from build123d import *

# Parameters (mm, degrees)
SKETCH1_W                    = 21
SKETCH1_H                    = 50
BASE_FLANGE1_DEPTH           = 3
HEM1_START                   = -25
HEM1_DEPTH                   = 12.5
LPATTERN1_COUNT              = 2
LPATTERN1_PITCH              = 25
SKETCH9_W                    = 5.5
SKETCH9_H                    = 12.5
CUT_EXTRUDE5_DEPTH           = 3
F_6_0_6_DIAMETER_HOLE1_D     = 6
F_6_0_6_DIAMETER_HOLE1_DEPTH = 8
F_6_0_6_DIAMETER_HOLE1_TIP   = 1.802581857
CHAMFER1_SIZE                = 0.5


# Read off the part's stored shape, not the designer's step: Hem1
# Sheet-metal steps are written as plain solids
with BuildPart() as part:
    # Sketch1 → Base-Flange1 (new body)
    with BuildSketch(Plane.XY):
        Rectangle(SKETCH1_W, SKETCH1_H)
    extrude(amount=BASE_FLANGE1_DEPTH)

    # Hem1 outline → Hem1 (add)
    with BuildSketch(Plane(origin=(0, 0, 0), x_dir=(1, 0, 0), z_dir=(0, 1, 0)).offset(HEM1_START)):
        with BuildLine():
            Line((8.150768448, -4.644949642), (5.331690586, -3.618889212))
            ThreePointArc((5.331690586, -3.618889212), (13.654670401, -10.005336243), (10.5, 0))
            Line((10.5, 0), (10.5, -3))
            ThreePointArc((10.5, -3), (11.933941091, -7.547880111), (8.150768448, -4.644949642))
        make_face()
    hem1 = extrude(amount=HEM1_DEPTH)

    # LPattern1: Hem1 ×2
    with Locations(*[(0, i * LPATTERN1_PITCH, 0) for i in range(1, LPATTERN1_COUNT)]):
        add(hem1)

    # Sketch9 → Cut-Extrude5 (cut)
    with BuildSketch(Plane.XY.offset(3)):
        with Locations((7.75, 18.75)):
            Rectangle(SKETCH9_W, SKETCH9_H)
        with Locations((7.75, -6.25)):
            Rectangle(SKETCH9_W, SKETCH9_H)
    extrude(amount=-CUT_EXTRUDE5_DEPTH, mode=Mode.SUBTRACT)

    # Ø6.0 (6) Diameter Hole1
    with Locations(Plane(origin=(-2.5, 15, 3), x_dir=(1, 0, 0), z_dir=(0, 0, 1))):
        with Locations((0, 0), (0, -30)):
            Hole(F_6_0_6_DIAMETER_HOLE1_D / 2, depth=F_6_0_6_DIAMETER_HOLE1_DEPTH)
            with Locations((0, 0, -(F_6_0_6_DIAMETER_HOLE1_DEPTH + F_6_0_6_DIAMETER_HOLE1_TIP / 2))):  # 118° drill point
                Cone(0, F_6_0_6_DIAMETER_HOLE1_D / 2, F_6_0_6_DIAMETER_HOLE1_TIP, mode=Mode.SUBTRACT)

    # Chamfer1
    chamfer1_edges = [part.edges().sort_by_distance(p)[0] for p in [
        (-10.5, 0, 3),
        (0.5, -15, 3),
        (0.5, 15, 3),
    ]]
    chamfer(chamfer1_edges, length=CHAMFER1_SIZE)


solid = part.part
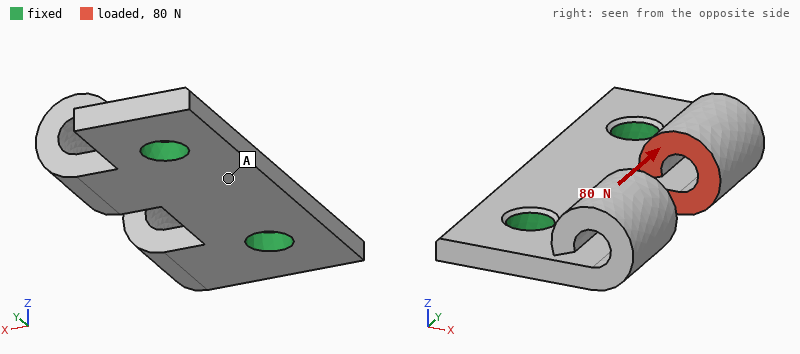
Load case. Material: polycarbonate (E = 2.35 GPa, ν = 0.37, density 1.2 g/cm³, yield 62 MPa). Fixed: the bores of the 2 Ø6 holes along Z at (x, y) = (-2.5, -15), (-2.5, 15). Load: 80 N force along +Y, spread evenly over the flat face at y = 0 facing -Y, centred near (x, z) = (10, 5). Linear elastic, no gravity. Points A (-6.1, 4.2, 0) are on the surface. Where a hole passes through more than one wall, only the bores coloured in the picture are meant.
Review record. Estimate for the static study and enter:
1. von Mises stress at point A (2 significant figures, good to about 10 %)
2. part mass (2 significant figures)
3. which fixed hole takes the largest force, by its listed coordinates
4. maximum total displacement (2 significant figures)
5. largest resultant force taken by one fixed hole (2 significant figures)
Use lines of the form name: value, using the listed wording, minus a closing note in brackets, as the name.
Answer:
von Mises stress at point A: 2.7 MPa
part mass: 4.9 g
which fixed hole takes the largest force, by its listed coordinates: (-2.5, 15)
maximum total displacement: 0.56 mm
largest resultant force taken by one fixed hole: 63 N
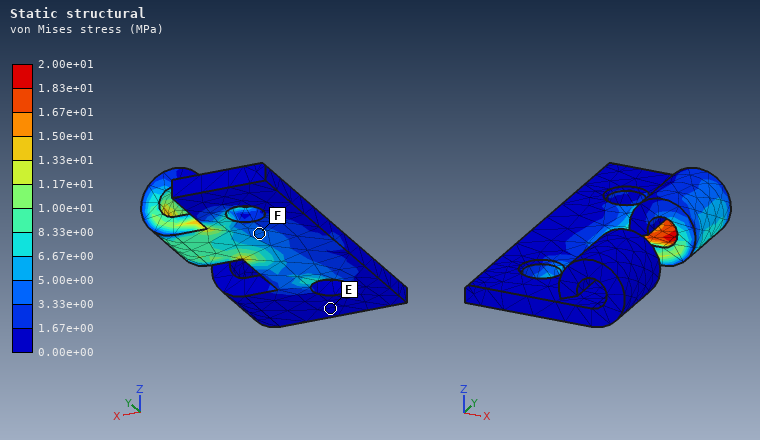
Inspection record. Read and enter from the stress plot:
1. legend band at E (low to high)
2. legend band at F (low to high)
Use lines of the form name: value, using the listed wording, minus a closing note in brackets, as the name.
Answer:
legend band at E: 0.00e+00 to 1.67e+00 MPa
legend band at F: 3.33e+00 to 5.00e+00 MPa
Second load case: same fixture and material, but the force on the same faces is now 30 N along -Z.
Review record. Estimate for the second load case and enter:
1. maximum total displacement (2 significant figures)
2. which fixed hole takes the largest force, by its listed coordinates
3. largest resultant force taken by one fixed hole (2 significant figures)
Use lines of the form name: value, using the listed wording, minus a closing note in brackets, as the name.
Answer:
maximum total displacement: 0.64 mm
which fixed hole takes the largest force, by its listed coordinates: (-2.5, 15)
largest resultant force taken by one fixed hole: 17 N
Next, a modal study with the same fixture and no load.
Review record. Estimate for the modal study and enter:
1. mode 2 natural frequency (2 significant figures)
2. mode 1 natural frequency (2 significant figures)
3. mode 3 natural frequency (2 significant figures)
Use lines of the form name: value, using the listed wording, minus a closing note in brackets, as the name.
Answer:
mode 2 natural frequency: 1300 Hz
mode 1 natural frequency: 1300 Hz
mode 3 natural frequency: 1900 Hz
